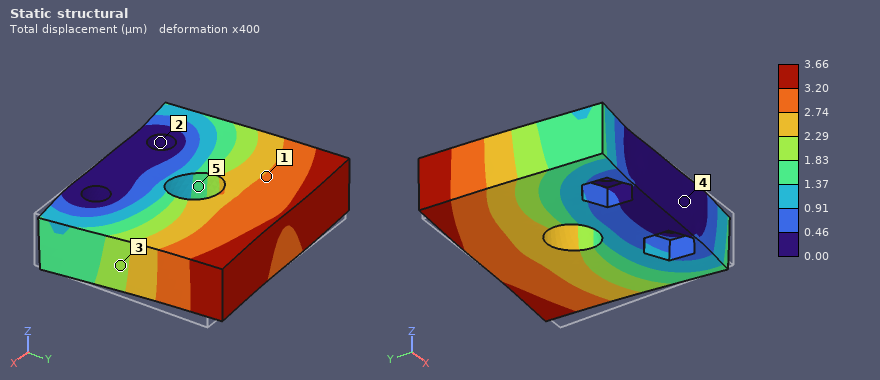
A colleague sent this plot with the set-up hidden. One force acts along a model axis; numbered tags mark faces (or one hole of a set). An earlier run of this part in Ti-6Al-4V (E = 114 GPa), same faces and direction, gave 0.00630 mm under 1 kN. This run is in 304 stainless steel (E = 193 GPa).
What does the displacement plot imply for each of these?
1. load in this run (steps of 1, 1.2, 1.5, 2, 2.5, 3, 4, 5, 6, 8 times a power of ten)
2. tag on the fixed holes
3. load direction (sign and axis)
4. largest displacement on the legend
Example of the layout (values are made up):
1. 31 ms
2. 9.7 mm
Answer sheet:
1. 1 kN
2. 2
3. -X
4. 3.66 µm
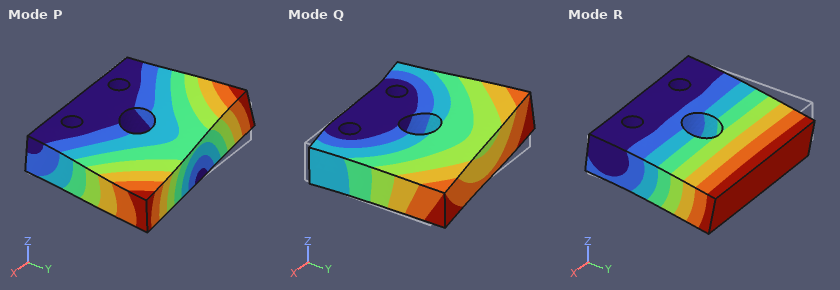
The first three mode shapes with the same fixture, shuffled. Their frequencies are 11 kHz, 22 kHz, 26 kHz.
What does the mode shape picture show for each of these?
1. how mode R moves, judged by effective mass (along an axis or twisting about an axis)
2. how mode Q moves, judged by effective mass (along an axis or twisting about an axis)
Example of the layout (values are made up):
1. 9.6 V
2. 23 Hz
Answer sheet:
1. along Z
2. along X
